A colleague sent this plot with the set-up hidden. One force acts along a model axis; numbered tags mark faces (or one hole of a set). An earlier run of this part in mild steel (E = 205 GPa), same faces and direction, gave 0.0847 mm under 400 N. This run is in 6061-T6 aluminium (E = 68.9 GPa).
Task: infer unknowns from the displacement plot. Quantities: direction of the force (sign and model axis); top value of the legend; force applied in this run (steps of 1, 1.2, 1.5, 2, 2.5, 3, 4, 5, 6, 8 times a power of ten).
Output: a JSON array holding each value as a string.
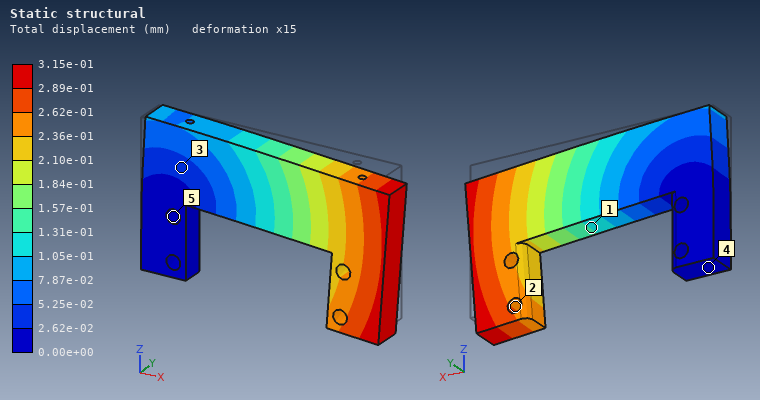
["-Z", "3.15e-01 mm", "500 N"]
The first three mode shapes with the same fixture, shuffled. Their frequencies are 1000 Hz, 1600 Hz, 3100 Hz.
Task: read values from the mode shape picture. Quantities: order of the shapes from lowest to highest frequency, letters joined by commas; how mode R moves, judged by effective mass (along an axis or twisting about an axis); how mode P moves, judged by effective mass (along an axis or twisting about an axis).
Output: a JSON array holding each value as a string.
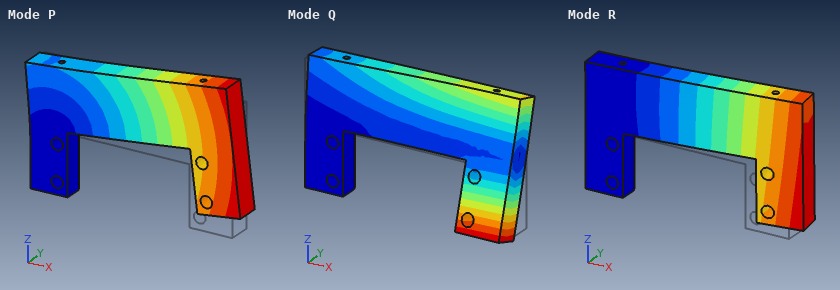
["R, P, Q", "along Y", "along Z"]
